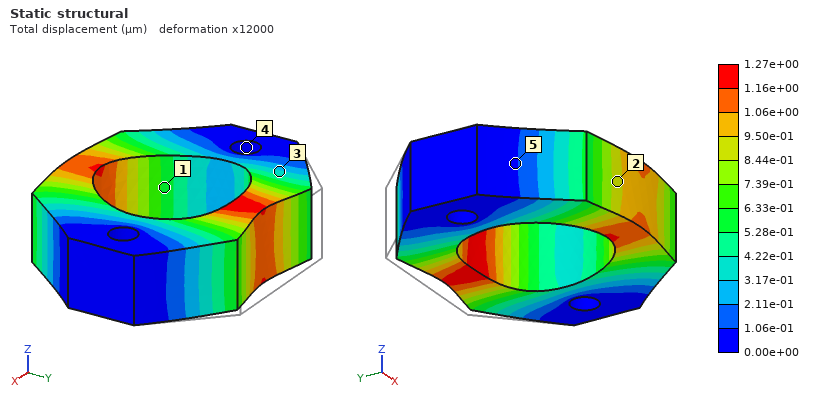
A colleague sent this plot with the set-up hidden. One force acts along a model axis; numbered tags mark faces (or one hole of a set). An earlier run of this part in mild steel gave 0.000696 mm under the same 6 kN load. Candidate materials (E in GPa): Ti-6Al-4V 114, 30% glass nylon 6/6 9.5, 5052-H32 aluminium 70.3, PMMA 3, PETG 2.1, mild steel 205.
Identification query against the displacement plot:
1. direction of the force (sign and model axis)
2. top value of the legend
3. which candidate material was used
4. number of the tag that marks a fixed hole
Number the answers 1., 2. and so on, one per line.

1. -Y
2. 1.27e+00 µm
3. Ti-6Al-4V
4. 4
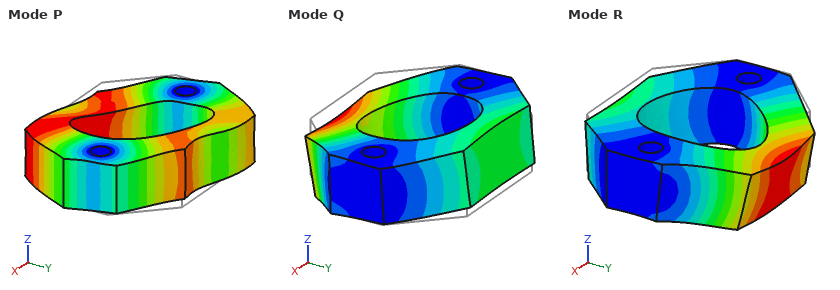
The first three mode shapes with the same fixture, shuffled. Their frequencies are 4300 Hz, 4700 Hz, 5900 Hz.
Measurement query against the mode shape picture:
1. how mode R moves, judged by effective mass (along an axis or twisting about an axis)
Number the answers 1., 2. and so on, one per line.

1. along Z
